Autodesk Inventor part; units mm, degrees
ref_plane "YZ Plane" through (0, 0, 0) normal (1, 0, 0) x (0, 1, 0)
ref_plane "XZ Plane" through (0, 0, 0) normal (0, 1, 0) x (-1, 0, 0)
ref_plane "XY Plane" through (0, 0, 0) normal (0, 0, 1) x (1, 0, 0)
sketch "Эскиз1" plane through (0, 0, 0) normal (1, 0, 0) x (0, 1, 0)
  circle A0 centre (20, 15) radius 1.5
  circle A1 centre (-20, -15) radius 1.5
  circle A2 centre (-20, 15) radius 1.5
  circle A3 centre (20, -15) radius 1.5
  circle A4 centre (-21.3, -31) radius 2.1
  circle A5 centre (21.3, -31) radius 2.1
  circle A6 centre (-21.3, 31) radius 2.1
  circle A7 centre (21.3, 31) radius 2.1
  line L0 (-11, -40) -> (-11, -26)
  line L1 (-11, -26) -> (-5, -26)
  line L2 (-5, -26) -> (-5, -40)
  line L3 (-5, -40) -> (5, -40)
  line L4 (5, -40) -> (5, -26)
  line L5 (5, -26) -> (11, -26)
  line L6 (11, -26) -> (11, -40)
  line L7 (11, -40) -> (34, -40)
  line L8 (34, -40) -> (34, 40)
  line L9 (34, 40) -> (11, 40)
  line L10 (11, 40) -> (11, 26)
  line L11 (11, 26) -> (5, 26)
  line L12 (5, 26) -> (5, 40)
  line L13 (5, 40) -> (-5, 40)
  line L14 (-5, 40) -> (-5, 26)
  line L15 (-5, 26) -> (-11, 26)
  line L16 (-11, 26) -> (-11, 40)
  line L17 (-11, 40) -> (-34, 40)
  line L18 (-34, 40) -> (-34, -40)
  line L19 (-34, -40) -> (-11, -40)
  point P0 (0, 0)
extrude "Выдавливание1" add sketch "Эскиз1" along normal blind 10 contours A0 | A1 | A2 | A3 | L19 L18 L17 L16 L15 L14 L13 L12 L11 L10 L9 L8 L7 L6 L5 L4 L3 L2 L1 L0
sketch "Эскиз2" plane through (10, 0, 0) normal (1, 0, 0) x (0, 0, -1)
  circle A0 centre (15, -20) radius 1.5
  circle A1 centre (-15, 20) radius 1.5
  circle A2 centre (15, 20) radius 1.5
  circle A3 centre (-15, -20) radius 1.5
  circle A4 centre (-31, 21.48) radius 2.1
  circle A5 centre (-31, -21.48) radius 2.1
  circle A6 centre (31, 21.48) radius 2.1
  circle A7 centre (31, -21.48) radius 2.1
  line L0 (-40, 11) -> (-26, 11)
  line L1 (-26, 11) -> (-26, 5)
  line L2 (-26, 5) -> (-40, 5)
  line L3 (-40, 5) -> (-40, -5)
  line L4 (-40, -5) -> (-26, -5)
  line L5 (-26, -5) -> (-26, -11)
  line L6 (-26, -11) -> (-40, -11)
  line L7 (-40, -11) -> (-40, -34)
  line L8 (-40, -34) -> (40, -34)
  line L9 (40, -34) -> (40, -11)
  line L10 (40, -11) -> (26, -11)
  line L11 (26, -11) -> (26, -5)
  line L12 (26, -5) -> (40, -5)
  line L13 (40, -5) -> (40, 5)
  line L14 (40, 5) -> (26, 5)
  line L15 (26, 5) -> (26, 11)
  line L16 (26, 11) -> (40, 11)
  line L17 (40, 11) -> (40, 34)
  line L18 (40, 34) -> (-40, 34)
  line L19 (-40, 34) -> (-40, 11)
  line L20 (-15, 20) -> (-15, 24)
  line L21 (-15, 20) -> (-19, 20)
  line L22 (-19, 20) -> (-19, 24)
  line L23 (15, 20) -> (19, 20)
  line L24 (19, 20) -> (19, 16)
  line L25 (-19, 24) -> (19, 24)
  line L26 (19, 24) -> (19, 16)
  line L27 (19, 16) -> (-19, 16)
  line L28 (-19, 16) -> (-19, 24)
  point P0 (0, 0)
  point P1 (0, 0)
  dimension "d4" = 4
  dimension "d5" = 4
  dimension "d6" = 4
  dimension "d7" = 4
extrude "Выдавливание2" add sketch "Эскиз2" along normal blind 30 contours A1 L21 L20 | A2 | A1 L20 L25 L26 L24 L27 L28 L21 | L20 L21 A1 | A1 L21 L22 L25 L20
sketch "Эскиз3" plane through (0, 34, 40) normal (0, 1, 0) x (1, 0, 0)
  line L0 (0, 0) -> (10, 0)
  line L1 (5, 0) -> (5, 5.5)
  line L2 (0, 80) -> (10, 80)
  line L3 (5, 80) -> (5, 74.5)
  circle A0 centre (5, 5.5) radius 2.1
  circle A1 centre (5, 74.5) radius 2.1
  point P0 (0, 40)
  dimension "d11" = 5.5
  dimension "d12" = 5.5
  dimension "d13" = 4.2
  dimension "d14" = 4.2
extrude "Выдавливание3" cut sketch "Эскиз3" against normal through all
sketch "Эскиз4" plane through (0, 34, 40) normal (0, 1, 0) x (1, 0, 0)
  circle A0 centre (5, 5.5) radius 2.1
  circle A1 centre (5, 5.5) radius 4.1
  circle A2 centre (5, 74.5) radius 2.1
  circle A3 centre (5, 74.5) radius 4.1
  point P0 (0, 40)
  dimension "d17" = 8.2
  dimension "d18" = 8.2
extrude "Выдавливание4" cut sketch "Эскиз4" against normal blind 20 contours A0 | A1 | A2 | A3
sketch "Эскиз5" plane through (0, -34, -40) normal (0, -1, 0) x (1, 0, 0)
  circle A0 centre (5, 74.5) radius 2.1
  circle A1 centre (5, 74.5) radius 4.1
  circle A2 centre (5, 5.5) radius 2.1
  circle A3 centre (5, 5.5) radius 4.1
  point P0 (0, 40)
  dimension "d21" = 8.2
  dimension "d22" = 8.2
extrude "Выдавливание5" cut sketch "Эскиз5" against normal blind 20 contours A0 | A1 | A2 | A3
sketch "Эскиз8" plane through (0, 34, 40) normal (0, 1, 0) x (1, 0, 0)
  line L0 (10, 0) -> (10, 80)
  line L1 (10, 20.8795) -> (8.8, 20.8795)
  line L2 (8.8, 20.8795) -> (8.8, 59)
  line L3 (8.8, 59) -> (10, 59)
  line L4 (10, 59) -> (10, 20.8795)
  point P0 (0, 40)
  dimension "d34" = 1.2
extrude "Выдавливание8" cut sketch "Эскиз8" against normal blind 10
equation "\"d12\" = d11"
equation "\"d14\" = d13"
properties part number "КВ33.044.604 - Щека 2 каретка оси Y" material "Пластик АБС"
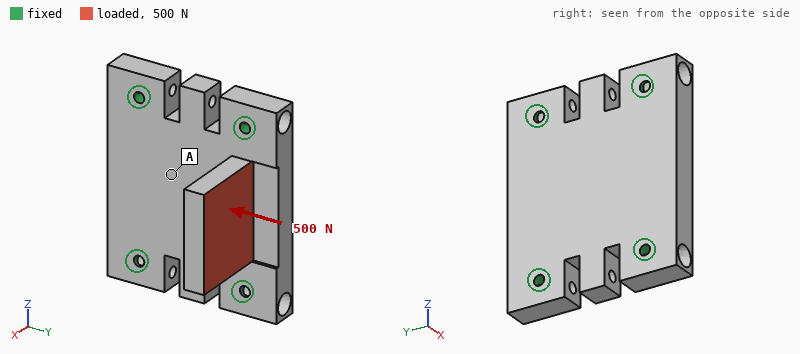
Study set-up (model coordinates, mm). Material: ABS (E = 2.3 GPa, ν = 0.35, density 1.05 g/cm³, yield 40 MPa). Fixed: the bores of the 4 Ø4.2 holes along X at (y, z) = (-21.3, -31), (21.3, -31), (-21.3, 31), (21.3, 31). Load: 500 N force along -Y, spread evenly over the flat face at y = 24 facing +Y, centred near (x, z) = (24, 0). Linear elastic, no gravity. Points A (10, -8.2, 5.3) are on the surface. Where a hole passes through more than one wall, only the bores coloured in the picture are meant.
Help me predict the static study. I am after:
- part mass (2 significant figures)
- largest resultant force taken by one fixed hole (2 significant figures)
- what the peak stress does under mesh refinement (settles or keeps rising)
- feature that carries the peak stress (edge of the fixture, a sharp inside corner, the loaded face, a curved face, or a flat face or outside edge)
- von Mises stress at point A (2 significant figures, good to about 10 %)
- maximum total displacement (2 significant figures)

57 g
160 N
keeps rising
a sharp inside corner
1.9 MPa
0.90 mm
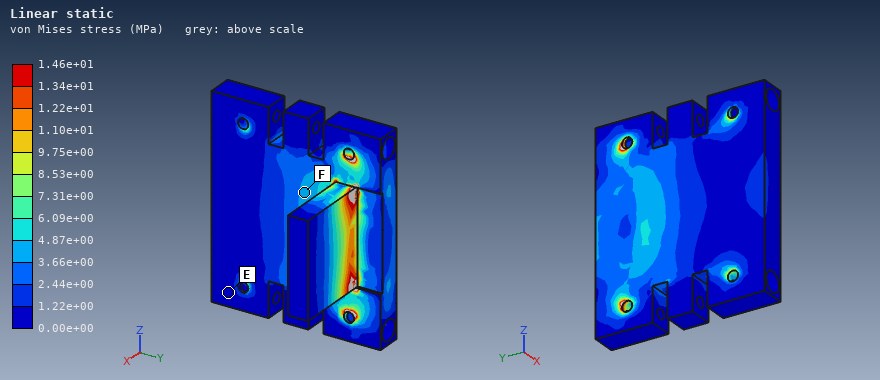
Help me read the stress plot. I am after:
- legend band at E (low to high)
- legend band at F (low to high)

0.00e+00 to 1.22e+00 MPa
3.66e+00 to 4.87e+00 MPa
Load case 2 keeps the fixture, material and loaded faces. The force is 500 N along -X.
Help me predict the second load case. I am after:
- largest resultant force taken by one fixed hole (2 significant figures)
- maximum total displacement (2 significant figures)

260 N
0.32 mm
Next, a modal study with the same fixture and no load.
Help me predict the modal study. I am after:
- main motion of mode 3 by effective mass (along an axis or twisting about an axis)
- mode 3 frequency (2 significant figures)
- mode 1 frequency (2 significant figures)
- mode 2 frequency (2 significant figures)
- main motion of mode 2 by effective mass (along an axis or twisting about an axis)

twisting about Z
3300 Hz
1400 Hz
2600 Hz
along X
